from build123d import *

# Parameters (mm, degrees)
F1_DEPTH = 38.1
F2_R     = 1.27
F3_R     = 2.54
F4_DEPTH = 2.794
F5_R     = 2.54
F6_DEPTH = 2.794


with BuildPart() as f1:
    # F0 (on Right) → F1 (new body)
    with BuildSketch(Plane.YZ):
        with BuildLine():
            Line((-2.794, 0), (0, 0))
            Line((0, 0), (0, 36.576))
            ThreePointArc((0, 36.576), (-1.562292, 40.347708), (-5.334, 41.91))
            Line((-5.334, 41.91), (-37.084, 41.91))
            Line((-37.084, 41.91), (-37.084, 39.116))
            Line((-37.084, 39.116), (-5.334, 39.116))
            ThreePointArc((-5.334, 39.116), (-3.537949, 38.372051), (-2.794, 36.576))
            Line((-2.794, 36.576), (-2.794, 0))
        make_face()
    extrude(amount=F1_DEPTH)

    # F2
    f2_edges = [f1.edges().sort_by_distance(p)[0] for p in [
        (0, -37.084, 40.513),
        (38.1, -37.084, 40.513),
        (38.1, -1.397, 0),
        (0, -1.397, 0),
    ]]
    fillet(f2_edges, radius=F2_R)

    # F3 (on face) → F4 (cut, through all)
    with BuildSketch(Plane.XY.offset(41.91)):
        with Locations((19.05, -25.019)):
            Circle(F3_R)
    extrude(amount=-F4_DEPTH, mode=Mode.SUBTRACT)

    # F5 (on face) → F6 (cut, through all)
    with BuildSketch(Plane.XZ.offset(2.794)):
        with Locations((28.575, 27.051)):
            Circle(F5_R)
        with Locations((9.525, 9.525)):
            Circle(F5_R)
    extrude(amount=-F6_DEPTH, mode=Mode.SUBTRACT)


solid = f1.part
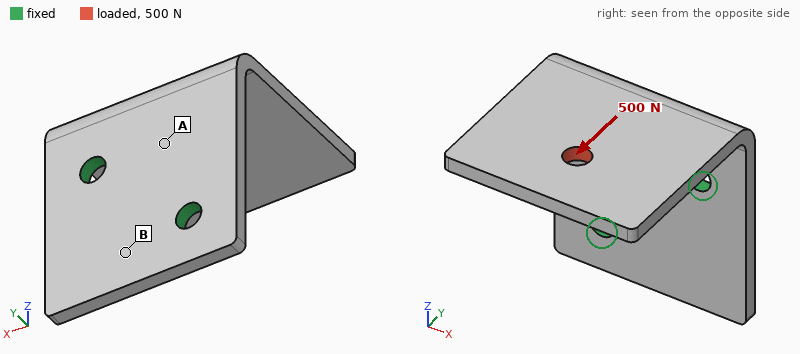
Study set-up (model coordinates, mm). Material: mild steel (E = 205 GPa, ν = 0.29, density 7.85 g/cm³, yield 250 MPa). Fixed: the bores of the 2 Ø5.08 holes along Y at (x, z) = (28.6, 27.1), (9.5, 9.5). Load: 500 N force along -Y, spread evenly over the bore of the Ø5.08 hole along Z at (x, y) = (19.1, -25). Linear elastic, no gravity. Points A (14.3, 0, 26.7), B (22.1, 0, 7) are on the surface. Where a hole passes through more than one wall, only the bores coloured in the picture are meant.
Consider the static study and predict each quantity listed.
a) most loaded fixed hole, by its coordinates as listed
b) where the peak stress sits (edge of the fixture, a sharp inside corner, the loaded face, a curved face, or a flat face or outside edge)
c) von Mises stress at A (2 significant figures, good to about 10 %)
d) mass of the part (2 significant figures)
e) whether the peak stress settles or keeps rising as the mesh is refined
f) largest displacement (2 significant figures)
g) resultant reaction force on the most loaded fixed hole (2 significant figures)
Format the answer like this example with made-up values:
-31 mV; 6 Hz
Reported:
(28.6, 27.1); edge of the fixture; 71 MPa; 61 g; keeps rising; 0.20 mm; 490 N
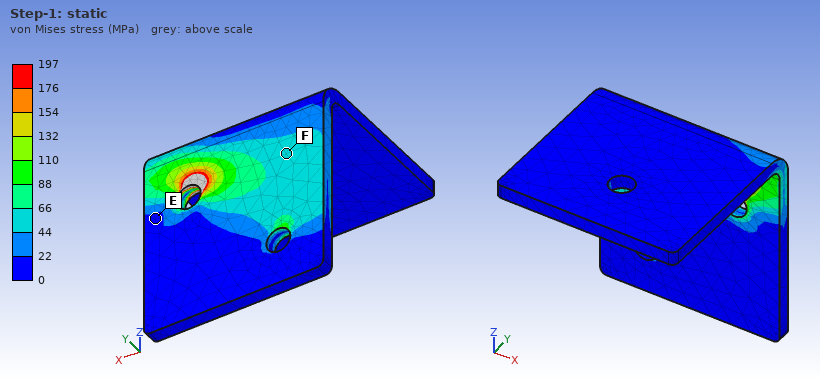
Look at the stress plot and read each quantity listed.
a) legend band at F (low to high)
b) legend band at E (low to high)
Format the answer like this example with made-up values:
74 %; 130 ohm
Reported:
44 to 66 MPa; 0 to 22 MPa
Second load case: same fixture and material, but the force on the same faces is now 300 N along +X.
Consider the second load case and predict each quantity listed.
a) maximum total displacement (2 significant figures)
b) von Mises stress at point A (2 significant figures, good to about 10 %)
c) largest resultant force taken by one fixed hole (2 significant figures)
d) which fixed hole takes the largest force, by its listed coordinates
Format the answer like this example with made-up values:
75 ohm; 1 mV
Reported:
0.17 mm; 58 MPa; 360 N; (28.6, 27.1)
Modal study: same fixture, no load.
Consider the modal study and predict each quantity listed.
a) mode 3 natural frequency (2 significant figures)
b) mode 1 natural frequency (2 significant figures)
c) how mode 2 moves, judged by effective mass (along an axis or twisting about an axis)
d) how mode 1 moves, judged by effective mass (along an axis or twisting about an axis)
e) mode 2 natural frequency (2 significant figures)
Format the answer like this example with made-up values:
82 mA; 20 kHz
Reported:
3700 Hz; 1100 Hz; along X; along Z; 1800 Hz
